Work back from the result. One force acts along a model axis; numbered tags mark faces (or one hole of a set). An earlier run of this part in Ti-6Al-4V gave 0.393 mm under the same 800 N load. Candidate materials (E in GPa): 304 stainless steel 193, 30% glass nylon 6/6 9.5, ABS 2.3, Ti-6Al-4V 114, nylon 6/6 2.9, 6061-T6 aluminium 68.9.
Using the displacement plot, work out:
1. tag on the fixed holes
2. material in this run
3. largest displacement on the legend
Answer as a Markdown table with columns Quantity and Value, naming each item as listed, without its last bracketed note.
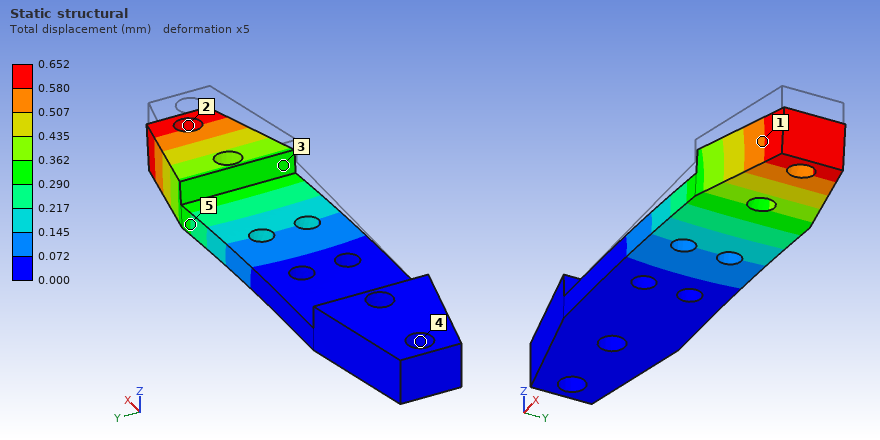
| Quantity | Value |
|---|---|
| tag on the fixed holes | 4 |
| material in this run | 6061-T6 aluminium |
| largest displacement on the legend | 0.652 mm |
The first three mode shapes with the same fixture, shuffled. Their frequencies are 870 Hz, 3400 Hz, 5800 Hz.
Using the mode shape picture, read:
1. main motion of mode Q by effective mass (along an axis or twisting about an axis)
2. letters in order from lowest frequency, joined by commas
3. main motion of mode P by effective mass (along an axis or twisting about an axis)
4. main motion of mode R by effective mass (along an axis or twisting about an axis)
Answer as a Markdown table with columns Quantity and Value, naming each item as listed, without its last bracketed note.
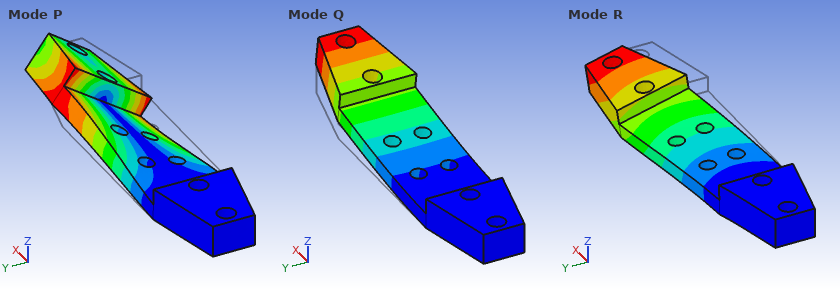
| Quantity | Value |
|---|---|
| main motion of mode Q by effective mass | along Z |
| letters in order from lowest frequency, joined by commas | Q, R, P |
| main motion of mode P by effective mass | twisting about X |
| main motion of mode R by effective mass | along Y |
